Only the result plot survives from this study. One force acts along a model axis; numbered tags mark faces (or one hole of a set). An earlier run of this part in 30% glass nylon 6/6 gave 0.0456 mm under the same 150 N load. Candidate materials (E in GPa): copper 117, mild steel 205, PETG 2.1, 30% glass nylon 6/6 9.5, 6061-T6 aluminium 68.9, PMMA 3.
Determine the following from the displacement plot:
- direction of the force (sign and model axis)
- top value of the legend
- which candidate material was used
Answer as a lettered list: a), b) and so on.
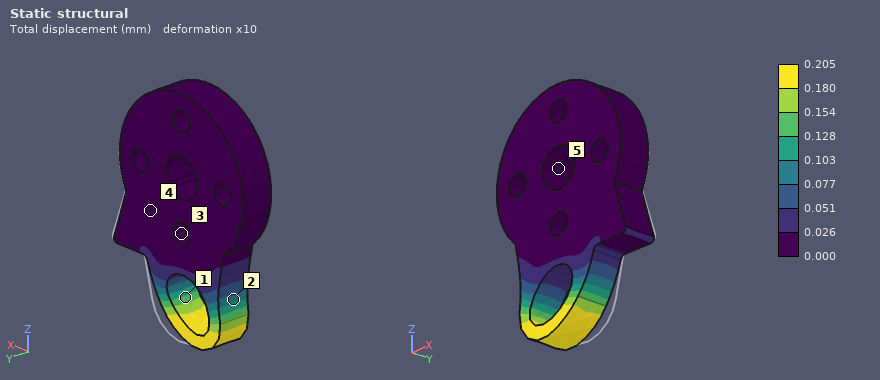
a) -X
b) 0.205 mm
c) PETG
